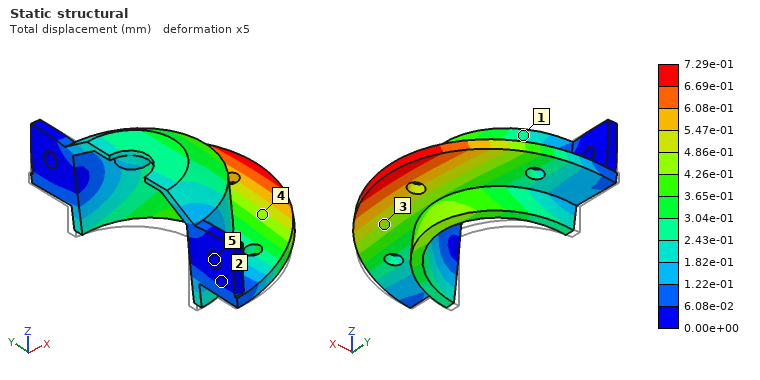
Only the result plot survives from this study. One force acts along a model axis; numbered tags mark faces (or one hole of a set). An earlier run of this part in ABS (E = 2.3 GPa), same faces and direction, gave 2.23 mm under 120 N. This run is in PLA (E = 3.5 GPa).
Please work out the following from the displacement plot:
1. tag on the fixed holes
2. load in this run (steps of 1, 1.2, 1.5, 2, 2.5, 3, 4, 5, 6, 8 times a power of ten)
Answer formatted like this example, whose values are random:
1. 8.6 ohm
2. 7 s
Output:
1. 5
2. 60 N
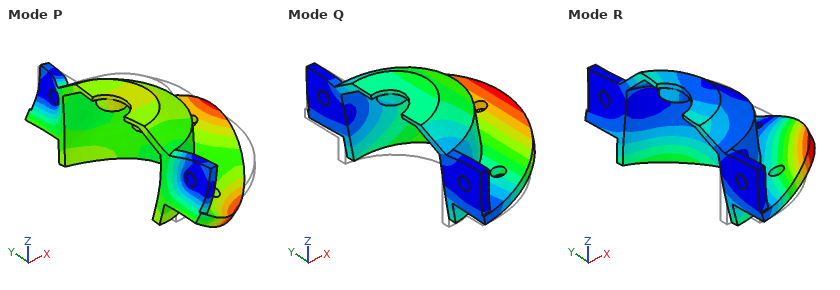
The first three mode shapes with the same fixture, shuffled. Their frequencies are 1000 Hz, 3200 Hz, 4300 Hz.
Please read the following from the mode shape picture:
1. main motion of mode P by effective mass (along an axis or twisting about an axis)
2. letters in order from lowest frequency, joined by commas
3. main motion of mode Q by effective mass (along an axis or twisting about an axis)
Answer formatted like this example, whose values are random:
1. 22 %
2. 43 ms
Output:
1. along X
2. Q, R, P
3. along Z
